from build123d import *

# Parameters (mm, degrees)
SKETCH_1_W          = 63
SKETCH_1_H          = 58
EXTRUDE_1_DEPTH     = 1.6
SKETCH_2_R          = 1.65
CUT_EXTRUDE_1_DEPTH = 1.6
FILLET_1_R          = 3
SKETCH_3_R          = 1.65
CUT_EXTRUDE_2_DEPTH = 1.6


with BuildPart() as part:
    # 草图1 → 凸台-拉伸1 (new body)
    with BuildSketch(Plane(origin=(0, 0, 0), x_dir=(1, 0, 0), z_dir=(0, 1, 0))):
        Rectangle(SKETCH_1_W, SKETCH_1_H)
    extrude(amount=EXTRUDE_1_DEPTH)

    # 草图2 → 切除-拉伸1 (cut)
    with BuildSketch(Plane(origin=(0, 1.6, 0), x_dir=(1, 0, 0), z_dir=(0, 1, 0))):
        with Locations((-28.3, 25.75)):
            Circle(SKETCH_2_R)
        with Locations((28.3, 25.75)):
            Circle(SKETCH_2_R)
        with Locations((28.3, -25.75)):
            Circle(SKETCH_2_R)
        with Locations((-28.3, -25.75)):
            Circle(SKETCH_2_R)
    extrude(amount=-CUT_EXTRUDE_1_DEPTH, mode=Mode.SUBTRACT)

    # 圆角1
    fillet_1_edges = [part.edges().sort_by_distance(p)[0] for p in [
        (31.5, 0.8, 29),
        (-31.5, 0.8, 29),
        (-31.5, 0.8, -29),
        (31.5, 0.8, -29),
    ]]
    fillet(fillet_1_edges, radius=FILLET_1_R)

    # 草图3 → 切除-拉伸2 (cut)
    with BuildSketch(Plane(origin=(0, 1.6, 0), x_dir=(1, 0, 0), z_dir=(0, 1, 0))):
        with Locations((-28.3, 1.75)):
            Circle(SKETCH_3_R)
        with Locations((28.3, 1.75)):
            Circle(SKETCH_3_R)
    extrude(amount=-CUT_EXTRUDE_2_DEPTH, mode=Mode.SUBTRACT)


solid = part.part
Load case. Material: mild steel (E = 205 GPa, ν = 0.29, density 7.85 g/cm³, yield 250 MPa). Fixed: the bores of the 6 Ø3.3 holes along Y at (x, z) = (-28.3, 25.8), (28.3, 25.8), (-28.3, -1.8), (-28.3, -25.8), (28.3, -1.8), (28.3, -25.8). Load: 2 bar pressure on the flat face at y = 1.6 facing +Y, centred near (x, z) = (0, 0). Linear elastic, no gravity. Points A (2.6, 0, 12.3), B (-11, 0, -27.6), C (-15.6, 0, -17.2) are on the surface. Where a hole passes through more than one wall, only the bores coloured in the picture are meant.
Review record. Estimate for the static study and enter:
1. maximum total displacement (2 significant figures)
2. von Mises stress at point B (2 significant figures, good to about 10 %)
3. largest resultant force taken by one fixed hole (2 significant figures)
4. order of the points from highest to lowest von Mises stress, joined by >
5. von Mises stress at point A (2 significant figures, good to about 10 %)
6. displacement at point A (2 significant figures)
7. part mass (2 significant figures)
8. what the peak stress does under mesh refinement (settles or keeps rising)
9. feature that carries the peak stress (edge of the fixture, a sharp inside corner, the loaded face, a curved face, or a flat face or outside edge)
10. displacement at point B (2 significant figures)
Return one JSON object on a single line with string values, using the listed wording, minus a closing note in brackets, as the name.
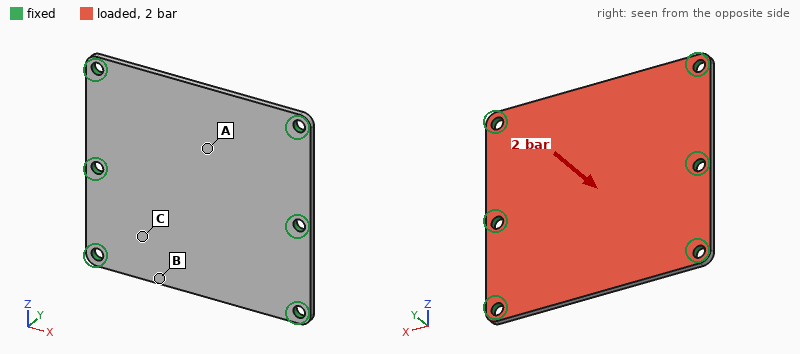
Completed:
{"maximum total displacement": "85 µm", "von Mises stress at point B": "41 MPa", "largest resultant force taken by one fixed hole": "170 N", "order of the points from highest to lowest von Mises stress, joined by >": "A > B > C", "von Mises stress at point A": "57 MPa", "displacement at point A": "84 µm", "part mass": "45 g", "what the peak stress does under mesh refinement": "keeps rising", "feature that carries the peak stress": "edge of the fixture", "displacement at point B": "58 µm"}
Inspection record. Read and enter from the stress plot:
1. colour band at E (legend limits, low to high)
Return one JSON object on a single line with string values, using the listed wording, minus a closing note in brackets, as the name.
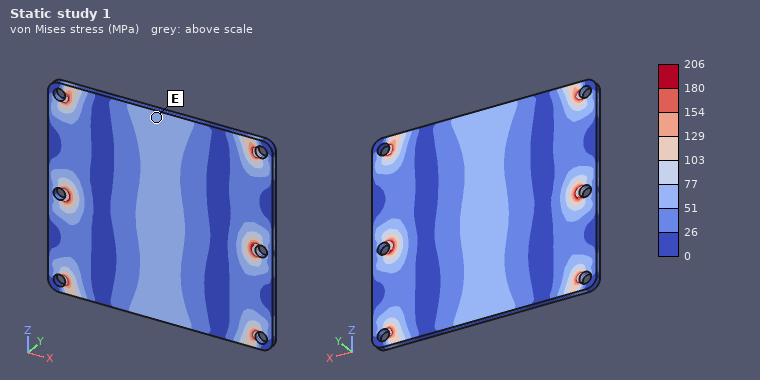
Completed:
{"colour band at E": "51 to 77 MPa"}
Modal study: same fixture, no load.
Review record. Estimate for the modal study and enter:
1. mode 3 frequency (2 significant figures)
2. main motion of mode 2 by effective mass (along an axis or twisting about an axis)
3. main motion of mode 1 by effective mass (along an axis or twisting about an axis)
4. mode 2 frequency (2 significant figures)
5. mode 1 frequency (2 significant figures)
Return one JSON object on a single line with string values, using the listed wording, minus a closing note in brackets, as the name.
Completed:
{"mode 3 frequency": "5200 Hz", "main motion of mode 2 by effective mass": "twisting about X", "main motion of mode 1 by effective mass": "along Y", "mode 2 frequency": "3100 Hz", "mode 1 frequency": "2500 Hz"}
